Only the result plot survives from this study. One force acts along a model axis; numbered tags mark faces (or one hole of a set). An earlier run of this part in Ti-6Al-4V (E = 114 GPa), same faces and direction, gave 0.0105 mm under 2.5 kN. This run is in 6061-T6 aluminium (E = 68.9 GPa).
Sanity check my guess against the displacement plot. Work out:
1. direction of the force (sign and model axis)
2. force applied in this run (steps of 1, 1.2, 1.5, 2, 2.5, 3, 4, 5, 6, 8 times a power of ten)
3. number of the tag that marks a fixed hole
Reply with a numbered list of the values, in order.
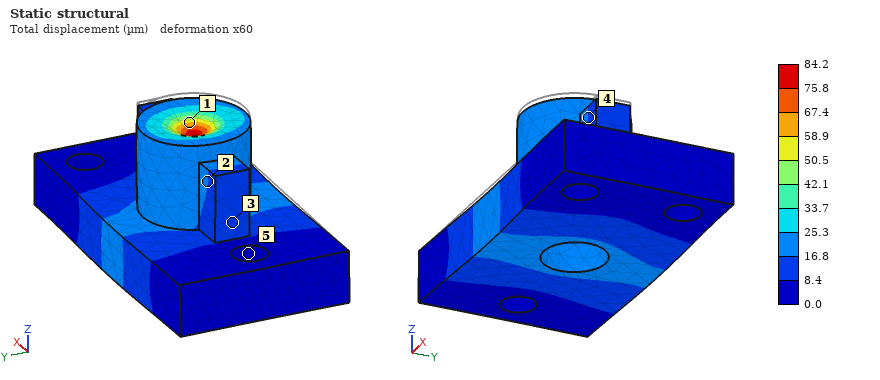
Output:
1. -Z
2. 12 kN
3. 5
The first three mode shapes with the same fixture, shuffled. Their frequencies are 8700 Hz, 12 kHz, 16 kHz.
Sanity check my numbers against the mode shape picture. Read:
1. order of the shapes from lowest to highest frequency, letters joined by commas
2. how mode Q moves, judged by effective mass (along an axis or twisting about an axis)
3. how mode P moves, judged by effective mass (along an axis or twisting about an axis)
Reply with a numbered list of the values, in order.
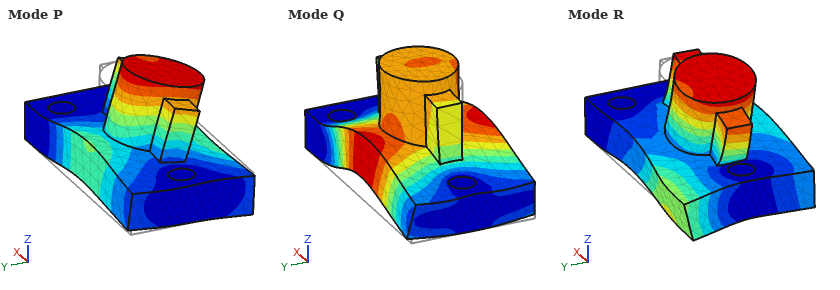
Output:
1. P, Q, R
2. along Z
3. along Y
